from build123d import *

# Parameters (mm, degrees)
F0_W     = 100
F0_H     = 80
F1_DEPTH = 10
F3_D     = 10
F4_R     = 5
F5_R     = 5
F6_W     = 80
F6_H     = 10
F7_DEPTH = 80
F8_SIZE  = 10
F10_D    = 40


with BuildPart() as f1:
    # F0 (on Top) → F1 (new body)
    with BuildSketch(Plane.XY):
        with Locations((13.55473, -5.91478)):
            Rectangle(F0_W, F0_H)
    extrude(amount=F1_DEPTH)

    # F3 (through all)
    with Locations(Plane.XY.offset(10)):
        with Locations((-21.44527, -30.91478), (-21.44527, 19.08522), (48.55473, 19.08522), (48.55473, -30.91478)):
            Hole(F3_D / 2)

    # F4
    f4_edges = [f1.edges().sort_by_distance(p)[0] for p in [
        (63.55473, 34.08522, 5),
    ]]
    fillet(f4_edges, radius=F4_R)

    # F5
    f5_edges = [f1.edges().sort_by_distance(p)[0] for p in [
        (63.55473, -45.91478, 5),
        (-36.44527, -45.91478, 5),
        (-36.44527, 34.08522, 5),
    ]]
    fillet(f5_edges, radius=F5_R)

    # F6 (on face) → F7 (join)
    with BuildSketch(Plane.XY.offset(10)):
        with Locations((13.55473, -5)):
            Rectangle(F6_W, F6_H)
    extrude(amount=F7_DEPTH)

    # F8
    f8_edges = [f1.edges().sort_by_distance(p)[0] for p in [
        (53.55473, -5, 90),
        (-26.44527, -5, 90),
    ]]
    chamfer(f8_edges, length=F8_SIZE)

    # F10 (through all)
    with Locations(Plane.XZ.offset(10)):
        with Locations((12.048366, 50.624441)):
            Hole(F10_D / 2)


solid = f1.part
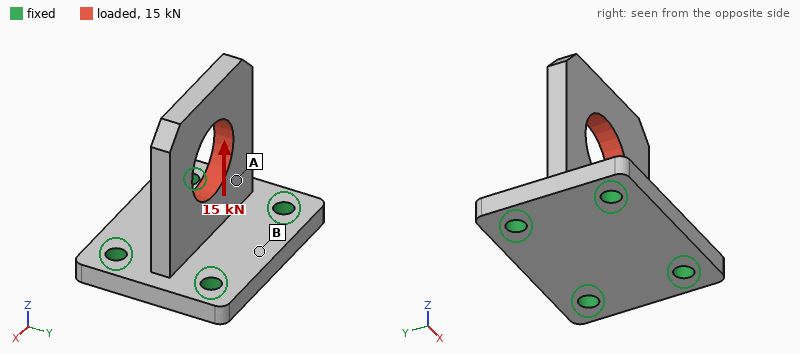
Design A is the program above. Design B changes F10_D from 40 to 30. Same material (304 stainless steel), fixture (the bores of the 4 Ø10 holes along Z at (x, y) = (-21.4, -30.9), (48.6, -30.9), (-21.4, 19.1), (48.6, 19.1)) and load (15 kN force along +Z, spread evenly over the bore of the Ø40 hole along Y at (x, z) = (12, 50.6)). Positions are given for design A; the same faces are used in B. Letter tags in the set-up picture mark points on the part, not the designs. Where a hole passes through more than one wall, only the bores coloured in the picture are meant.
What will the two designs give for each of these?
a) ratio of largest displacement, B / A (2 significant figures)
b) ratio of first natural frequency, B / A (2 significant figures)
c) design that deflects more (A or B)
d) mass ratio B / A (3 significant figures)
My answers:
0.87
1.0
A
1.04
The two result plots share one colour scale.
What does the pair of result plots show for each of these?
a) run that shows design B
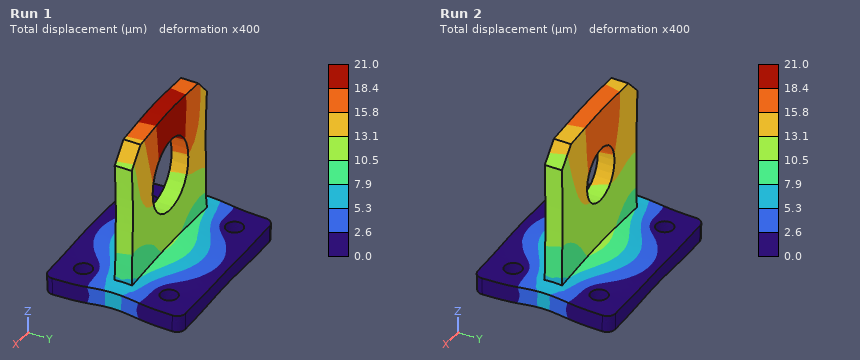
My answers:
Run 2
